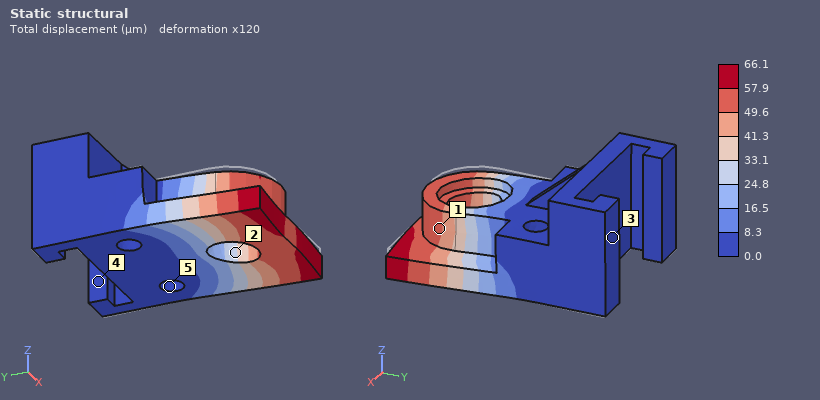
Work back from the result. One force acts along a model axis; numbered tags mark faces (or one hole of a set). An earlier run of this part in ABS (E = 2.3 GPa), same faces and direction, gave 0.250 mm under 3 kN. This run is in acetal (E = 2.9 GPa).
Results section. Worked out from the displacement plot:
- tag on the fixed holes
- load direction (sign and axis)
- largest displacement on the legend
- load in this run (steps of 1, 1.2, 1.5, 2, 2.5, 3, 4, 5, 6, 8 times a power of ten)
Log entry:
5
+X
66.1 µm
1 kN
